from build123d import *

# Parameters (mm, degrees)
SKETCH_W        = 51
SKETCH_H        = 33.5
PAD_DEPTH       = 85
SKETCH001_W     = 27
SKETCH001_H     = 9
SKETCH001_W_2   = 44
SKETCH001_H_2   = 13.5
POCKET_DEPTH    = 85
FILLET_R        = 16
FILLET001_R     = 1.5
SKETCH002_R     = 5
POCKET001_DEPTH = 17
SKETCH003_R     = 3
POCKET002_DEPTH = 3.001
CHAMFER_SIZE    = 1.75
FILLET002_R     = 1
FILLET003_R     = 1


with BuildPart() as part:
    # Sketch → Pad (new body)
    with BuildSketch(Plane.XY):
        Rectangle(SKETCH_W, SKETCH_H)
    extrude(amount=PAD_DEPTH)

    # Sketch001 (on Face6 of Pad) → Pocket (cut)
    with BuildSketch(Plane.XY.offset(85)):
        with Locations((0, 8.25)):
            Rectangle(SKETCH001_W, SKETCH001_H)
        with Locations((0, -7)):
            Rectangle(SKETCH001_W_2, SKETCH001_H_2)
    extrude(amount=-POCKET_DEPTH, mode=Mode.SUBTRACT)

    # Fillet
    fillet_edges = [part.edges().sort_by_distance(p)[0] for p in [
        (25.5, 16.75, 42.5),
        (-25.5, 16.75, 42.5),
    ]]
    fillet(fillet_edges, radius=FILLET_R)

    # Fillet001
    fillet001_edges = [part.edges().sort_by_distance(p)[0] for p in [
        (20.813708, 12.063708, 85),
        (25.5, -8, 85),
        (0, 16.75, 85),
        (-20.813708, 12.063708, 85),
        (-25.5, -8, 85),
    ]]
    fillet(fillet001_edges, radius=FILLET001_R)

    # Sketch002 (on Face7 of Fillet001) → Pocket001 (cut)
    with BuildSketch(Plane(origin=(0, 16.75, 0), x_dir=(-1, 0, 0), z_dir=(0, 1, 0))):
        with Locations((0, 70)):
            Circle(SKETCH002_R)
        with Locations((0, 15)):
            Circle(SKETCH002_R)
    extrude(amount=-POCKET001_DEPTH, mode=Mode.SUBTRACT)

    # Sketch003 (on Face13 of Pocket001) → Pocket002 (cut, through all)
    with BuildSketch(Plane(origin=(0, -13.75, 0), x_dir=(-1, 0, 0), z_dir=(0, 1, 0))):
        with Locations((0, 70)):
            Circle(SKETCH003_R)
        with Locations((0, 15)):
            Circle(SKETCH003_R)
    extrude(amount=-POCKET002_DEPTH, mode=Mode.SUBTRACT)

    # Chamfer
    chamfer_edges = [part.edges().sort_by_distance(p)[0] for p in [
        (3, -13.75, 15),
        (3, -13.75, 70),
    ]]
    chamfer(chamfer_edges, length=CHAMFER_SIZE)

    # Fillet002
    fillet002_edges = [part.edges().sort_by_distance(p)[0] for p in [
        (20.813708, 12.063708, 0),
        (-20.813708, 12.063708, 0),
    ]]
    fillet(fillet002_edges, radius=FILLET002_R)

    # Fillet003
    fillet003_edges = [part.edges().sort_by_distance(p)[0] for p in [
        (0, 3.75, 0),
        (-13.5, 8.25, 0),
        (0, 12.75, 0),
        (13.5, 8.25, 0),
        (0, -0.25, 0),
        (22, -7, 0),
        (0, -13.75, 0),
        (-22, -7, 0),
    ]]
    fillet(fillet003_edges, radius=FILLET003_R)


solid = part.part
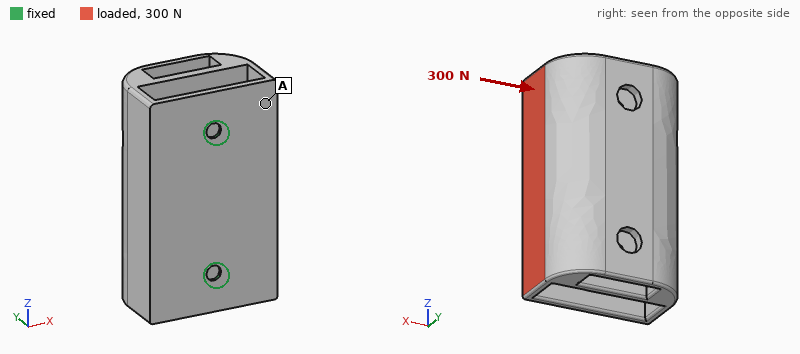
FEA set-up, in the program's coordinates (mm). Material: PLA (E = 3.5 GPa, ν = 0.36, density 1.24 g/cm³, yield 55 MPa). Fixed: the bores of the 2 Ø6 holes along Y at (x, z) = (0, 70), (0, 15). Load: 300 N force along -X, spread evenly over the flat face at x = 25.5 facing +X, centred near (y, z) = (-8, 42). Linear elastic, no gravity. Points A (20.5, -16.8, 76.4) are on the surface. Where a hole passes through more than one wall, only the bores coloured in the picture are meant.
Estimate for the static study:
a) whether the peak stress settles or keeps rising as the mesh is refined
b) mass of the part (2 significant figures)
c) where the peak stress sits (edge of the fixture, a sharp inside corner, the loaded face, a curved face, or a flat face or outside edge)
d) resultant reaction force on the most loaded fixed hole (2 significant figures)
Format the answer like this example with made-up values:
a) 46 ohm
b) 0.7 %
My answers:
a) keeps rising
b) 78 g
c) edge of the fixture
d) 150 N
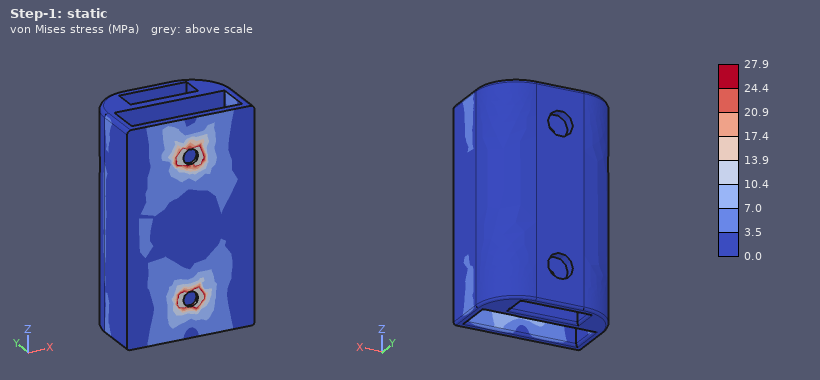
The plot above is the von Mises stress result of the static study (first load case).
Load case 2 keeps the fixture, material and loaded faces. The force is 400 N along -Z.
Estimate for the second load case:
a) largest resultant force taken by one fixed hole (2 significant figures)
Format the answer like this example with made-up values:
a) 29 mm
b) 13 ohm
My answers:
a) 270 N
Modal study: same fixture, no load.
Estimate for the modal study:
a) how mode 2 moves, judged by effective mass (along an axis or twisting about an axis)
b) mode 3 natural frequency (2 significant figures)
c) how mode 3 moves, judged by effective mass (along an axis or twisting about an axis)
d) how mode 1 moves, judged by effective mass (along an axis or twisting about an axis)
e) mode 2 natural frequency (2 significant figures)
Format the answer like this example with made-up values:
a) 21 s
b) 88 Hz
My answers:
a) along Z
b) 550 Hz
c) along Y
d) along X
e) 480 Hz
